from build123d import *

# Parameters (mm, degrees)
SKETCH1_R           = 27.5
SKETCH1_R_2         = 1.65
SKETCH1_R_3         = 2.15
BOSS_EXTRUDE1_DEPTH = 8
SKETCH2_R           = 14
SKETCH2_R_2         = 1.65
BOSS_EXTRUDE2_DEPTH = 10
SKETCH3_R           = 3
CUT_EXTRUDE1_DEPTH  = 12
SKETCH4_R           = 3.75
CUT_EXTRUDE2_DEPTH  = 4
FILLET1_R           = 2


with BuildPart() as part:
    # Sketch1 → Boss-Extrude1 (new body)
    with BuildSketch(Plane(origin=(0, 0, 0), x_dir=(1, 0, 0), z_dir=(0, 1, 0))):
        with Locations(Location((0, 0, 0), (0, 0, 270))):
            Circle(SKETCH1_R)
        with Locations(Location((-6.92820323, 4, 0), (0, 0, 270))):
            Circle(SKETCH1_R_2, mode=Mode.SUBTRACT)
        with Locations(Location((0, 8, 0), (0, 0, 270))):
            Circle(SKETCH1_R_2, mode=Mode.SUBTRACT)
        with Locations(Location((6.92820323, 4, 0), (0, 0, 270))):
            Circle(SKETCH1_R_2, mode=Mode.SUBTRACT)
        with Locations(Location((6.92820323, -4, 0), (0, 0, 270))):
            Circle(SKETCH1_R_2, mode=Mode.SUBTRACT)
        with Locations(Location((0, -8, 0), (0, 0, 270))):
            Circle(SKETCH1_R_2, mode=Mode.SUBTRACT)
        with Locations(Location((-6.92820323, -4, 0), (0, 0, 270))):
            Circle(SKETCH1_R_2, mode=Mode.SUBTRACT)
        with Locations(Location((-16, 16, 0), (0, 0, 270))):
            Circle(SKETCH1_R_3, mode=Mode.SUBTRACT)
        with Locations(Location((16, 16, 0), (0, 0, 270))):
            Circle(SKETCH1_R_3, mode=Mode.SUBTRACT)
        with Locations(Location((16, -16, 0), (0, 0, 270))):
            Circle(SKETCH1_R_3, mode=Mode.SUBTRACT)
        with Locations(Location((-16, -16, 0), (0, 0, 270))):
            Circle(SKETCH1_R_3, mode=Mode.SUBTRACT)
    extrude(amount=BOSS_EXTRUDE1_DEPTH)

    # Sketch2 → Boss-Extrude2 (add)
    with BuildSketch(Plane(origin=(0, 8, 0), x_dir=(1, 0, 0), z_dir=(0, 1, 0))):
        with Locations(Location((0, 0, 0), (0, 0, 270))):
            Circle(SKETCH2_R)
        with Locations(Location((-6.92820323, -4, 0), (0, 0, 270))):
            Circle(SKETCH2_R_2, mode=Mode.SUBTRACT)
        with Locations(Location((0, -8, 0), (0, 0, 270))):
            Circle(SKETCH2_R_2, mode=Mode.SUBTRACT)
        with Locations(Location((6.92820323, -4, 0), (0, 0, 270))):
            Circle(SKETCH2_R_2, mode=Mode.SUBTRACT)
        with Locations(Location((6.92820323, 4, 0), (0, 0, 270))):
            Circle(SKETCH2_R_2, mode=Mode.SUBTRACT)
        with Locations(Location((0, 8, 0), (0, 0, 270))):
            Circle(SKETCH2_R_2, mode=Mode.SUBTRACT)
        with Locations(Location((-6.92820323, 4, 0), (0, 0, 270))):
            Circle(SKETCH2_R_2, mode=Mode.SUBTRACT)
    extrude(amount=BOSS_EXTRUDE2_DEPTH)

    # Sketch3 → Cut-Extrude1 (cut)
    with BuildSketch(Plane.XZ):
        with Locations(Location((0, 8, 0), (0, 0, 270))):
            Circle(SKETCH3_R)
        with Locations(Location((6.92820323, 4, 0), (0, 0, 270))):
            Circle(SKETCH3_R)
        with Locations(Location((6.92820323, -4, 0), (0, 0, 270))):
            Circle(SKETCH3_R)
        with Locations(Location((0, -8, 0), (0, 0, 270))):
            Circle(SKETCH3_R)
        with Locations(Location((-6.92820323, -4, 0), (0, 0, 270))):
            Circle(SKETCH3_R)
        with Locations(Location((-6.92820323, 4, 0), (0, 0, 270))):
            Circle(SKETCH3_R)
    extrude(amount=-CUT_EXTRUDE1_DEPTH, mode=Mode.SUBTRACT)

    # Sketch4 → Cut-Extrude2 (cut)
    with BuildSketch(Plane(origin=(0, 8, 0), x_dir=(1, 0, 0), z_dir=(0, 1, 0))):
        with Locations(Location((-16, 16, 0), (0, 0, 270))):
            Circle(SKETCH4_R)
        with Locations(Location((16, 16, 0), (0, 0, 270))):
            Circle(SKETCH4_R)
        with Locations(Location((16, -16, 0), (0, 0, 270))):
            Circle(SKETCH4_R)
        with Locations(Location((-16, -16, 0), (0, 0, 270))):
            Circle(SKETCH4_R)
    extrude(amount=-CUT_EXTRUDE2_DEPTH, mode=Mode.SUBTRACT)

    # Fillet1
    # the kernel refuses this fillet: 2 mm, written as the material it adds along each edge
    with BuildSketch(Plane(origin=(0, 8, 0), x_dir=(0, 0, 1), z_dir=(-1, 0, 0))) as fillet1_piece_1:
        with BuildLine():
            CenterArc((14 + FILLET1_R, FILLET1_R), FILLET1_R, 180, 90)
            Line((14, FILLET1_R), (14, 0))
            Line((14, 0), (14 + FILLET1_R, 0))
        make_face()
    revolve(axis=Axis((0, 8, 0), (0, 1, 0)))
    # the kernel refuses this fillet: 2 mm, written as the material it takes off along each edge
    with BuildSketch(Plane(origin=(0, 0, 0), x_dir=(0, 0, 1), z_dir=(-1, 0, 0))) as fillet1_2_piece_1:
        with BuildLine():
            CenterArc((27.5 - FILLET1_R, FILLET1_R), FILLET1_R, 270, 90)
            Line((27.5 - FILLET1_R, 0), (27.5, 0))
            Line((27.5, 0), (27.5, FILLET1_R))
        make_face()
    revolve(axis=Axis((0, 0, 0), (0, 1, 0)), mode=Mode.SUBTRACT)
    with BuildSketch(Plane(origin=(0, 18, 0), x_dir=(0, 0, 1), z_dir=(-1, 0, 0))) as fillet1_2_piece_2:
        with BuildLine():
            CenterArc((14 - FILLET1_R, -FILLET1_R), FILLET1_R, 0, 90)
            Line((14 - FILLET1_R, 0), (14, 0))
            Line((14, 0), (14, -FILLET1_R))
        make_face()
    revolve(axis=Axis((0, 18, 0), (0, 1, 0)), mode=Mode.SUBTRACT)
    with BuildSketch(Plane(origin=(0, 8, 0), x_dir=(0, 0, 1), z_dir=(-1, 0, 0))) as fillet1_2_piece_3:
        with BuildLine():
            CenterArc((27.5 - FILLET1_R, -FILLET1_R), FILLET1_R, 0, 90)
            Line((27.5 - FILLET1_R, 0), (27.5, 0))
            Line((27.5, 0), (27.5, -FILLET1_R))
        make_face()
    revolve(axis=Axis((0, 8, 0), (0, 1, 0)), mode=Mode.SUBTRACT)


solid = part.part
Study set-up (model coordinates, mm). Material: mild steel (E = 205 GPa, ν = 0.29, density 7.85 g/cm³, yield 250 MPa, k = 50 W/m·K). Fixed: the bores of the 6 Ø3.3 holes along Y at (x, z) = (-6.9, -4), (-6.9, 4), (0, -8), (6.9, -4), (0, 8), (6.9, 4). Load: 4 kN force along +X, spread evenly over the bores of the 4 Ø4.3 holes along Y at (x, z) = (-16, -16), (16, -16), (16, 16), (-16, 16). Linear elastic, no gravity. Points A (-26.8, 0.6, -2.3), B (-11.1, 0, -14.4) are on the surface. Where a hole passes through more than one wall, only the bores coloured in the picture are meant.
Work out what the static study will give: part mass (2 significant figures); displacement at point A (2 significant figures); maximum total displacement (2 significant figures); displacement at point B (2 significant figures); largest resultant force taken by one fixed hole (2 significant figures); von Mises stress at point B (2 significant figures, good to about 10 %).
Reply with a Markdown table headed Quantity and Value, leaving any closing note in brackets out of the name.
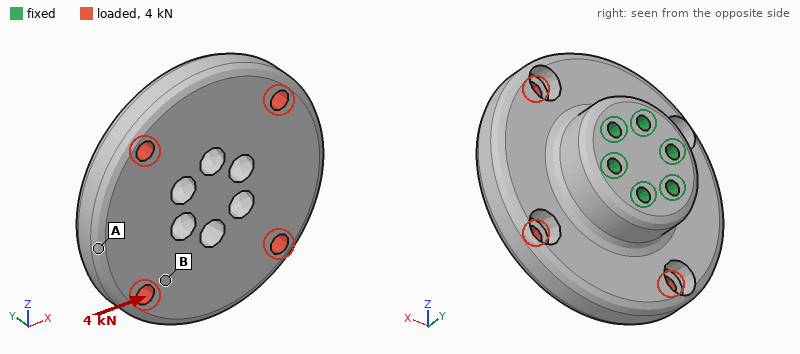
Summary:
| Quantity | Value |
|---|---|
| part mass | 170 g |
| displacement at point A | 7.3 µm |
| maximum total displacement | 7.3 µm |
| displacement at point B | 5.0 µm |
| largest resultant force taken by one fixed hole | 1.4 kN |
| von Mises stress at point B | 19 MPa |
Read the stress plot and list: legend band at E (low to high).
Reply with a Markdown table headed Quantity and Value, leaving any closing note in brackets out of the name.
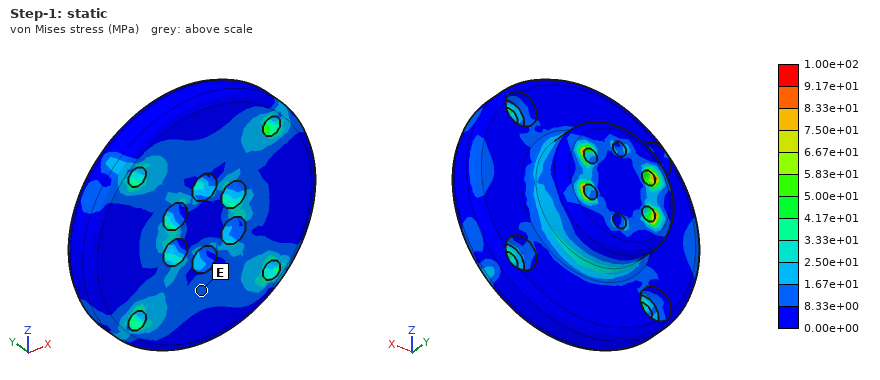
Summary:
| Quantity | Value |
|---|---|
| legend band at E | 8.33e+00 to 1.67e+01 MPa |
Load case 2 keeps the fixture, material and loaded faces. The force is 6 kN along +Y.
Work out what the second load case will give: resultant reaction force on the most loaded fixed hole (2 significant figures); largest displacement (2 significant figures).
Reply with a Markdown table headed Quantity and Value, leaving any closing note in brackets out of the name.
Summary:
| Quantity | Value |
|---|---|
| resultant reaction force on the most loaded fixed hole | 1.1 kN |
| largest displacement | 9.9 µm |
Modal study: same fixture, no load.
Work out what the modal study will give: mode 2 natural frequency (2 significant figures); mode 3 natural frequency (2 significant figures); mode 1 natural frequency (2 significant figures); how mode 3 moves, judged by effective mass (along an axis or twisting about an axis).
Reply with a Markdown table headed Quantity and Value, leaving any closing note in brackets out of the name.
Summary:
| Quantity | Value |
|---|---|
| mode 2 natural frequency | 11 kHz |
| mode 3 natural frequency | 13 kHz |
| mode 1 natural frequency | 11 kHz |
| how mode 3 moves, judged by effective mass | twisting about Y |
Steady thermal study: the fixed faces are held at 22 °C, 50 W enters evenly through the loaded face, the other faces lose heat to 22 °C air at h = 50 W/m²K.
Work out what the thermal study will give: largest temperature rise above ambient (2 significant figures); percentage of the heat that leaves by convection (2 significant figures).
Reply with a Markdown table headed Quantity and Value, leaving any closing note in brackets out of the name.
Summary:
| Quantity | Value |
|---|---|
| largest temperature rise above ambient | 47 K |
| percentage of the heat that leaves by convection | 17 % |
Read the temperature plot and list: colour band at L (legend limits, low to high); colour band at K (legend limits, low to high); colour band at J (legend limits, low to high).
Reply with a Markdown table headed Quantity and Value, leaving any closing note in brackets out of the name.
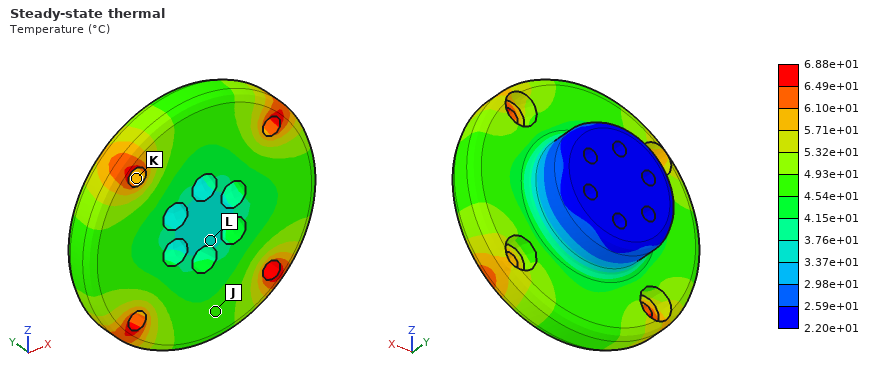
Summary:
| Quantity | Value |
|---|---|
| colour band at L | 3.37e+01 to 3.76e+01 °C |
| colour band at K | 5.71e+01 to 6.10e+01 °C |
| colour band at J | 4.54e+01 to 4.93e+01 °C |
